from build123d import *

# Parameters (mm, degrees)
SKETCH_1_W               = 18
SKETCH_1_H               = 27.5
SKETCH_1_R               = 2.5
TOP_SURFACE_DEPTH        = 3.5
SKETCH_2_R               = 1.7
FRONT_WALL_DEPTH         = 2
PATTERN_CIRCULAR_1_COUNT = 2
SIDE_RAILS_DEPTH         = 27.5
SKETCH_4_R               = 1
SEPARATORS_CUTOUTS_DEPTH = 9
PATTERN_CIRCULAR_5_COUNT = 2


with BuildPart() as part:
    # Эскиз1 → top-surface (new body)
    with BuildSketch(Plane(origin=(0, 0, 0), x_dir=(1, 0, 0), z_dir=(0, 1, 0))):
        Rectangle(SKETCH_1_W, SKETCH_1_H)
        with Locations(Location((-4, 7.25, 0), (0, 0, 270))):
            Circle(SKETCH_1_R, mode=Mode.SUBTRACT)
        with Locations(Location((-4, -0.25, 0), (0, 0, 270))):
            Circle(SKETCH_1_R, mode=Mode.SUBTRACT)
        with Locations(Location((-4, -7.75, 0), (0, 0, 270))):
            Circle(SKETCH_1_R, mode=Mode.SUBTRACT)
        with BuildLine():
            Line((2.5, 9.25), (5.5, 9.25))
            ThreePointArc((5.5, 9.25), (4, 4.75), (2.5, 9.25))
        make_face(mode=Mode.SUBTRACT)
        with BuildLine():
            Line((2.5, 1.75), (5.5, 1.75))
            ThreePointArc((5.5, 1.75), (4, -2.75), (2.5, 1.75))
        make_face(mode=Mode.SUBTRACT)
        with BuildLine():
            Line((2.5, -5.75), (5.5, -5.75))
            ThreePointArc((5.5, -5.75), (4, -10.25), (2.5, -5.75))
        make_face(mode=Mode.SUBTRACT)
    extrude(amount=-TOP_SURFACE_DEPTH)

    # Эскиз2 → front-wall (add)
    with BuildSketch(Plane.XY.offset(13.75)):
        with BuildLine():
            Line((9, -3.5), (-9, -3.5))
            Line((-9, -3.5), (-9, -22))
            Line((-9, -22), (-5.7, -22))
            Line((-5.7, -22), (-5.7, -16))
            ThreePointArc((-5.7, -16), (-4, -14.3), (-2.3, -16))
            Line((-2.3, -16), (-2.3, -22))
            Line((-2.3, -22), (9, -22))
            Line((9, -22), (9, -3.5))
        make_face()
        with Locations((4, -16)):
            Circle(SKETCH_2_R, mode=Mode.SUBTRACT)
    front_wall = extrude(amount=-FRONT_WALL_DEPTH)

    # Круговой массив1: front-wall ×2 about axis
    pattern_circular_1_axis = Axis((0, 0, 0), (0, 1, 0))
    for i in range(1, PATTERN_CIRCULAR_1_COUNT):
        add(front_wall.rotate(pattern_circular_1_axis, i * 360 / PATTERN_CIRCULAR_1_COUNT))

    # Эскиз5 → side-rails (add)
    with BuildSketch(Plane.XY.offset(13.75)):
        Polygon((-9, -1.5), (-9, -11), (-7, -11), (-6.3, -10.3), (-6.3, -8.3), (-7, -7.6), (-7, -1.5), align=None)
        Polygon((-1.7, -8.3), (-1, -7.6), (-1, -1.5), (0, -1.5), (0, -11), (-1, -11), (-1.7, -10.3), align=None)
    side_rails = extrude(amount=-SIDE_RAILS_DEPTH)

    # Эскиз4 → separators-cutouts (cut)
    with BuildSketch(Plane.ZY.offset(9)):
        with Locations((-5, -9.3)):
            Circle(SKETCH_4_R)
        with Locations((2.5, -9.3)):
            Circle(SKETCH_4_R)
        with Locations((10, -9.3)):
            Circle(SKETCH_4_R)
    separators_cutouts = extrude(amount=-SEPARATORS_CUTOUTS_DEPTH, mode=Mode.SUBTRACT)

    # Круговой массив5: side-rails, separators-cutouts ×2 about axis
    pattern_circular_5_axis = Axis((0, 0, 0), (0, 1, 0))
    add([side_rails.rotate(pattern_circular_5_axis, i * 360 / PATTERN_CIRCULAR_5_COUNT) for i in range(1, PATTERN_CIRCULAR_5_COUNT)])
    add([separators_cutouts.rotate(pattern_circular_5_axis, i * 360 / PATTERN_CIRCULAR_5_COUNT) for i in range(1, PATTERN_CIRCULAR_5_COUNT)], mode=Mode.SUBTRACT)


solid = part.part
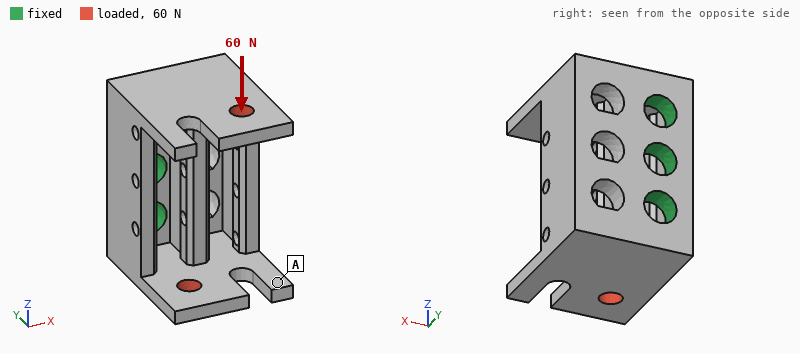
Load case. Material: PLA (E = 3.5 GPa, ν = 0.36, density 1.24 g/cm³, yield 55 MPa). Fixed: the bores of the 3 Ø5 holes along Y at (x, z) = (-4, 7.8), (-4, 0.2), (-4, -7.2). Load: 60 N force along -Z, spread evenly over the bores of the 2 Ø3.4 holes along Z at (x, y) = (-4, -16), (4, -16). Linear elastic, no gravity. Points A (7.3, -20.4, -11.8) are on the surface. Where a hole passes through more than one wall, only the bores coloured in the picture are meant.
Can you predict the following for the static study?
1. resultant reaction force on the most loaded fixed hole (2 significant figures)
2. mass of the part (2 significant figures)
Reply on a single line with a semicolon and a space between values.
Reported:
44 N; 4.6 g
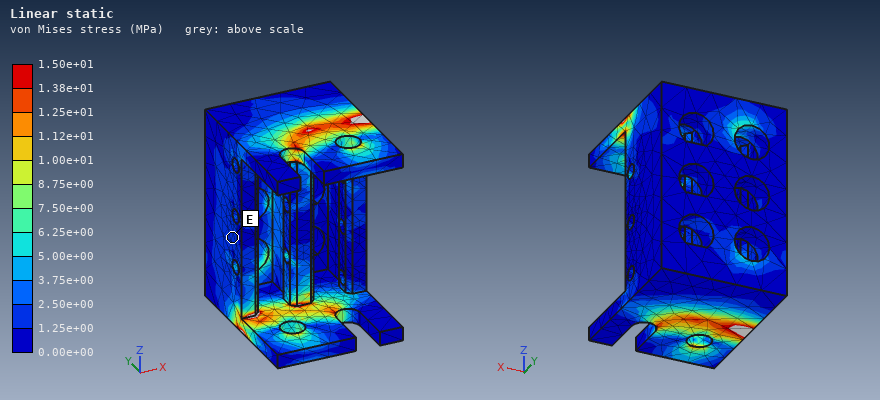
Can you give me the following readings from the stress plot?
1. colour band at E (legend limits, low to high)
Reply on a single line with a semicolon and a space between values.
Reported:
1.25e+00 to 2.50e+00 MPa
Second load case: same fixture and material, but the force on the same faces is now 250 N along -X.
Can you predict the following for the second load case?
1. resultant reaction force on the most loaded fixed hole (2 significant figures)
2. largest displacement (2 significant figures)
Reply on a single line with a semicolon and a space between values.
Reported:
140 N; 0.41 mm
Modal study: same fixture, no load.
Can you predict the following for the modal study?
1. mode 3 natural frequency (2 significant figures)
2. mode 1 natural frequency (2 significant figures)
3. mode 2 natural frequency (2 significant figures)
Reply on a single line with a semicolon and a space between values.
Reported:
3700 Hz; 3200 Hz; 3400 Hz
